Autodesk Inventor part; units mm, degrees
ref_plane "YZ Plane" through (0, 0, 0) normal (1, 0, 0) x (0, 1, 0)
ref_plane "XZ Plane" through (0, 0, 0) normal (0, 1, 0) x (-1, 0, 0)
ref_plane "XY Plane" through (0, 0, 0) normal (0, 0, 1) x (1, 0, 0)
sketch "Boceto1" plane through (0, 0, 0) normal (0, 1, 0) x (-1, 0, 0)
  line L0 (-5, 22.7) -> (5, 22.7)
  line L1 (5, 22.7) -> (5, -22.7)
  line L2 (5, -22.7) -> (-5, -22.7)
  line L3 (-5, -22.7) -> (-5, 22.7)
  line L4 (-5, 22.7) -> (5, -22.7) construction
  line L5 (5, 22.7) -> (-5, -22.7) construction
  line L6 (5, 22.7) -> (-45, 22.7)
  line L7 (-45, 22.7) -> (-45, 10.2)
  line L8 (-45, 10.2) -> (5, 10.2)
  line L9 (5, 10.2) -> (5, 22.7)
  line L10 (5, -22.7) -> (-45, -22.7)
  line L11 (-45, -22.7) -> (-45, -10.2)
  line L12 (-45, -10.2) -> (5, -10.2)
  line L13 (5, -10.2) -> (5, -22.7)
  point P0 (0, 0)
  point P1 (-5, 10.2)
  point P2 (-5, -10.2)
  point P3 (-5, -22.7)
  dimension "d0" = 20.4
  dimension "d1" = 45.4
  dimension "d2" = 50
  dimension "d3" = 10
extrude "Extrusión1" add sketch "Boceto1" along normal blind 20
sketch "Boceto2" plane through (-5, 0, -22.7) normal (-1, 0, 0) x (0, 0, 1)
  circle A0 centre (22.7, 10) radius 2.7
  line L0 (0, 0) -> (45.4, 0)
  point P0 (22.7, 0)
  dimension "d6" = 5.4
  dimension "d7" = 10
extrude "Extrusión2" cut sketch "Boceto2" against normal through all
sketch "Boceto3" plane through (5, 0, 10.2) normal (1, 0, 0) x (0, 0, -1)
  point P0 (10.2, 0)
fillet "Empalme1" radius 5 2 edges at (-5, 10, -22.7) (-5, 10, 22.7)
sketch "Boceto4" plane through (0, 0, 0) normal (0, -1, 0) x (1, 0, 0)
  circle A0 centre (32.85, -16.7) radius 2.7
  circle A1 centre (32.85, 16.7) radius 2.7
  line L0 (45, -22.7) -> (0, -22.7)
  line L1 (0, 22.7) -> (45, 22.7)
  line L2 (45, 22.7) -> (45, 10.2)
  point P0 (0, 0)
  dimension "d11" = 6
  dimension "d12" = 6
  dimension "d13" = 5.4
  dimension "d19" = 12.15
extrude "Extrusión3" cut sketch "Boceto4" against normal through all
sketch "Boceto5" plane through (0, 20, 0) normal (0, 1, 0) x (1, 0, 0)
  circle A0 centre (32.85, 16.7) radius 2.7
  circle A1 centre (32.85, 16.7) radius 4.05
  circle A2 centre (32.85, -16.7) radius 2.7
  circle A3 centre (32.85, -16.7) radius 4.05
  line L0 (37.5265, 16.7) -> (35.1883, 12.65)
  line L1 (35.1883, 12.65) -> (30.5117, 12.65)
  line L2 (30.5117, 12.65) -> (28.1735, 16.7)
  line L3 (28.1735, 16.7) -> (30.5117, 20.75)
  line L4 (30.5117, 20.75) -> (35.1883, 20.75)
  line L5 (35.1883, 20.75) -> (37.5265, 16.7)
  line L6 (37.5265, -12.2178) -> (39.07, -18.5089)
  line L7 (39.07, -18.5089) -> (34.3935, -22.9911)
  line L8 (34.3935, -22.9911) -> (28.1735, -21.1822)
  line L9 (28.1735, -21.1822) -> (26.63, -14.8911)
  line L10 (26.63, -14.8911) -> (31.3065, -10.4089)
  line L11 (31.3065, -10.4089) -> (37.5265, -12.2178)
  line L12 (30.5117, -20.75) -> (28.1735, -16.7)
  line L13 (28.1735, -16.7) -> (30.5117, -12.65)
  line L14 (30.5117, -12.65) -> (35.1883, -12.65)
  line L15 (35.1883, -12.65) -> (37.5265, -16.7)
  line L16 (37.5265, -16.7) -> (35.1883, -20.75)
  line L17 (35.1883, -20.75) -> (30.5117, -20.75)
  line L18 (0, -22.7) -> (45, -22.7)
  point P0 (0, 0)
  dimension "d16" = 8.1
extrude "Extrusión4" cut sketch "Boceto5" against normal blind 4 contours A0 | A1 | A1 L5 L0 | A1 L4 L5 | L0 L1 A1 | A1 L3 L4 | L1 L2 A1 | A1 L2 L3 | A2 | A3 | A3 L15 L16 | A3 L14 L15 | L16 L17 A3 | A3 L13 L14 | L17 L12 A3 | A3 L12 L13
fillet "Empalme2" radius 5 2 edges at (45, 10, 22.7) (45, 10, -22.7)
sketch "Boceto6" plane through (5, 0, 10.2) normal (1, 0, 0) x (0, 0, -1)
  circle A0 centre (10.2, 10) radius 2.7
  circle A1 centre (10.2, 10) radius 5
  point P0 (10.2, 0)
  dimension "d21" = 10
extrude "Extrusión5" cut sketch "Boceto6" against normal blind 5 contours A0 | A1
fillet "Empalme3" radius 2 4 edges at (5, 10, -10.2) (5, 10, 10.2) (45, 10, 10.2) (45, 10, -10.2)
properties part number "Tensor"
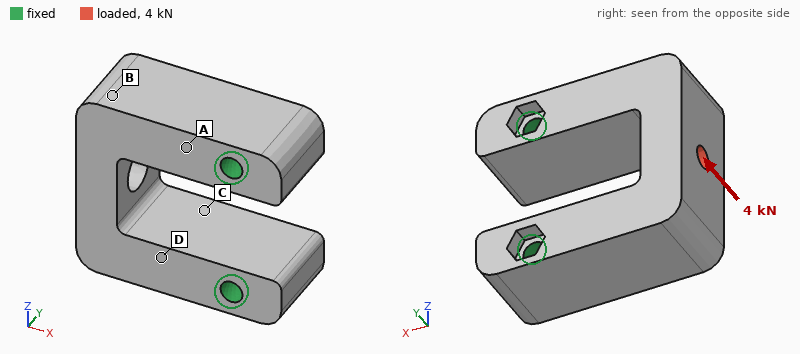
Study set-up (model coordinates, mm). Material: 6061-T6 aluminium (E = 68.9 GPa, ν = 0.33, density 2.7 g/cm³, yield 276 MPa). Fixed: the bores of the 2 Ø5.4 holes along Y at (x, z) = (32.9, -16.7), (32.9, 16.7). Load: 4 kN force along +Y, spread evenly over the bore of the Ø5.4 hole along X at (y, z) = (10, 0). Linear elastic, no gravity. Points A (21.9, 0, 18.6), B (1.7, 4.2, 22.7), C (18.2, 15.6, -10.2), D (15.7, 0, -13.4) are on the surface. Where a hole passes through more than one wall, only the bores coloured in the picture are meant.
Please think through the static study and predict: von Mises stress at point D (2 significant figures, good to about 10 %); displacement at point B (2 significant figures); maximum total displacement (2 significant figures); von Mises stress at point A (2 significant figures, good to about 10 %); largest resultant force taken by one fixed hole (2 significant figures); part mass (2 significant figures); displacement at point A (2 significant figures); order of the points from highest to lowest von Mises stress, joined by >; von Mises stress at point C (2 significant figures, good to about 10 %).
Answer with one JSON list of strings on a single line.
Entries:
["46 MPa", "61 µm", "99 µm", "67 MPa", "2.0 kN", "73 g", "19 µm", "A > D > C > B", "35 MPa"]
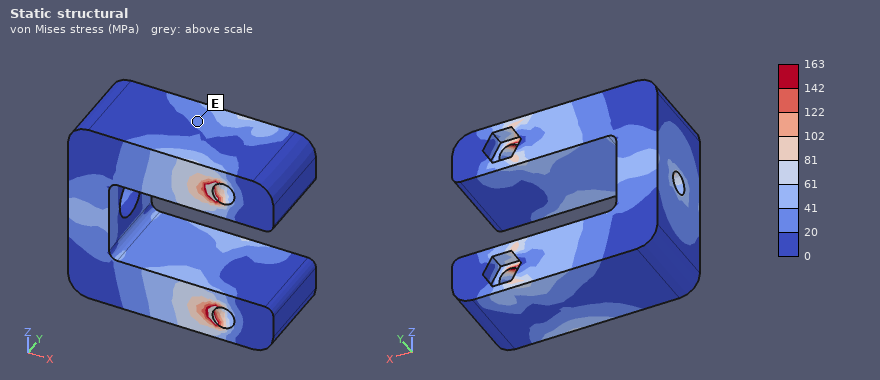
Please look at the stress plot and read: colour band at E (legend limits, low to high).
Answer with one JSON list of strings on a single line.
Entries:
["20 to 41 MPa"]
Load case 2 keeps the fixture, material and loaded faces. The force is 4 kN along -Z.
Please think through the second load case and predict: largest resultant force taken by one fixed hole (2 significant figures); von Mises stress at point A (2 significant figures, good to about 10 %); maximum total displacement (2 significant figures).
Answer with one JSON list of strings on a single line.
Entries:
["3.0 kN", "29 MPa", "63 µm"]
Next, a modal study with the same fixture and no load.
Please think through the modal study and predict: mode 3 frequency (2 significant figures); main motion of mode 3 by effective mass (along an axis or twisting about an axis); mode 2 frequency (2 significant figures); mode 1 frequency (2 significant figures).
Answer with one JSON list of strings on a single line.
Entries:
["11 kHz", "twisting about X", "7400 Hz", "7200 Hz"]
